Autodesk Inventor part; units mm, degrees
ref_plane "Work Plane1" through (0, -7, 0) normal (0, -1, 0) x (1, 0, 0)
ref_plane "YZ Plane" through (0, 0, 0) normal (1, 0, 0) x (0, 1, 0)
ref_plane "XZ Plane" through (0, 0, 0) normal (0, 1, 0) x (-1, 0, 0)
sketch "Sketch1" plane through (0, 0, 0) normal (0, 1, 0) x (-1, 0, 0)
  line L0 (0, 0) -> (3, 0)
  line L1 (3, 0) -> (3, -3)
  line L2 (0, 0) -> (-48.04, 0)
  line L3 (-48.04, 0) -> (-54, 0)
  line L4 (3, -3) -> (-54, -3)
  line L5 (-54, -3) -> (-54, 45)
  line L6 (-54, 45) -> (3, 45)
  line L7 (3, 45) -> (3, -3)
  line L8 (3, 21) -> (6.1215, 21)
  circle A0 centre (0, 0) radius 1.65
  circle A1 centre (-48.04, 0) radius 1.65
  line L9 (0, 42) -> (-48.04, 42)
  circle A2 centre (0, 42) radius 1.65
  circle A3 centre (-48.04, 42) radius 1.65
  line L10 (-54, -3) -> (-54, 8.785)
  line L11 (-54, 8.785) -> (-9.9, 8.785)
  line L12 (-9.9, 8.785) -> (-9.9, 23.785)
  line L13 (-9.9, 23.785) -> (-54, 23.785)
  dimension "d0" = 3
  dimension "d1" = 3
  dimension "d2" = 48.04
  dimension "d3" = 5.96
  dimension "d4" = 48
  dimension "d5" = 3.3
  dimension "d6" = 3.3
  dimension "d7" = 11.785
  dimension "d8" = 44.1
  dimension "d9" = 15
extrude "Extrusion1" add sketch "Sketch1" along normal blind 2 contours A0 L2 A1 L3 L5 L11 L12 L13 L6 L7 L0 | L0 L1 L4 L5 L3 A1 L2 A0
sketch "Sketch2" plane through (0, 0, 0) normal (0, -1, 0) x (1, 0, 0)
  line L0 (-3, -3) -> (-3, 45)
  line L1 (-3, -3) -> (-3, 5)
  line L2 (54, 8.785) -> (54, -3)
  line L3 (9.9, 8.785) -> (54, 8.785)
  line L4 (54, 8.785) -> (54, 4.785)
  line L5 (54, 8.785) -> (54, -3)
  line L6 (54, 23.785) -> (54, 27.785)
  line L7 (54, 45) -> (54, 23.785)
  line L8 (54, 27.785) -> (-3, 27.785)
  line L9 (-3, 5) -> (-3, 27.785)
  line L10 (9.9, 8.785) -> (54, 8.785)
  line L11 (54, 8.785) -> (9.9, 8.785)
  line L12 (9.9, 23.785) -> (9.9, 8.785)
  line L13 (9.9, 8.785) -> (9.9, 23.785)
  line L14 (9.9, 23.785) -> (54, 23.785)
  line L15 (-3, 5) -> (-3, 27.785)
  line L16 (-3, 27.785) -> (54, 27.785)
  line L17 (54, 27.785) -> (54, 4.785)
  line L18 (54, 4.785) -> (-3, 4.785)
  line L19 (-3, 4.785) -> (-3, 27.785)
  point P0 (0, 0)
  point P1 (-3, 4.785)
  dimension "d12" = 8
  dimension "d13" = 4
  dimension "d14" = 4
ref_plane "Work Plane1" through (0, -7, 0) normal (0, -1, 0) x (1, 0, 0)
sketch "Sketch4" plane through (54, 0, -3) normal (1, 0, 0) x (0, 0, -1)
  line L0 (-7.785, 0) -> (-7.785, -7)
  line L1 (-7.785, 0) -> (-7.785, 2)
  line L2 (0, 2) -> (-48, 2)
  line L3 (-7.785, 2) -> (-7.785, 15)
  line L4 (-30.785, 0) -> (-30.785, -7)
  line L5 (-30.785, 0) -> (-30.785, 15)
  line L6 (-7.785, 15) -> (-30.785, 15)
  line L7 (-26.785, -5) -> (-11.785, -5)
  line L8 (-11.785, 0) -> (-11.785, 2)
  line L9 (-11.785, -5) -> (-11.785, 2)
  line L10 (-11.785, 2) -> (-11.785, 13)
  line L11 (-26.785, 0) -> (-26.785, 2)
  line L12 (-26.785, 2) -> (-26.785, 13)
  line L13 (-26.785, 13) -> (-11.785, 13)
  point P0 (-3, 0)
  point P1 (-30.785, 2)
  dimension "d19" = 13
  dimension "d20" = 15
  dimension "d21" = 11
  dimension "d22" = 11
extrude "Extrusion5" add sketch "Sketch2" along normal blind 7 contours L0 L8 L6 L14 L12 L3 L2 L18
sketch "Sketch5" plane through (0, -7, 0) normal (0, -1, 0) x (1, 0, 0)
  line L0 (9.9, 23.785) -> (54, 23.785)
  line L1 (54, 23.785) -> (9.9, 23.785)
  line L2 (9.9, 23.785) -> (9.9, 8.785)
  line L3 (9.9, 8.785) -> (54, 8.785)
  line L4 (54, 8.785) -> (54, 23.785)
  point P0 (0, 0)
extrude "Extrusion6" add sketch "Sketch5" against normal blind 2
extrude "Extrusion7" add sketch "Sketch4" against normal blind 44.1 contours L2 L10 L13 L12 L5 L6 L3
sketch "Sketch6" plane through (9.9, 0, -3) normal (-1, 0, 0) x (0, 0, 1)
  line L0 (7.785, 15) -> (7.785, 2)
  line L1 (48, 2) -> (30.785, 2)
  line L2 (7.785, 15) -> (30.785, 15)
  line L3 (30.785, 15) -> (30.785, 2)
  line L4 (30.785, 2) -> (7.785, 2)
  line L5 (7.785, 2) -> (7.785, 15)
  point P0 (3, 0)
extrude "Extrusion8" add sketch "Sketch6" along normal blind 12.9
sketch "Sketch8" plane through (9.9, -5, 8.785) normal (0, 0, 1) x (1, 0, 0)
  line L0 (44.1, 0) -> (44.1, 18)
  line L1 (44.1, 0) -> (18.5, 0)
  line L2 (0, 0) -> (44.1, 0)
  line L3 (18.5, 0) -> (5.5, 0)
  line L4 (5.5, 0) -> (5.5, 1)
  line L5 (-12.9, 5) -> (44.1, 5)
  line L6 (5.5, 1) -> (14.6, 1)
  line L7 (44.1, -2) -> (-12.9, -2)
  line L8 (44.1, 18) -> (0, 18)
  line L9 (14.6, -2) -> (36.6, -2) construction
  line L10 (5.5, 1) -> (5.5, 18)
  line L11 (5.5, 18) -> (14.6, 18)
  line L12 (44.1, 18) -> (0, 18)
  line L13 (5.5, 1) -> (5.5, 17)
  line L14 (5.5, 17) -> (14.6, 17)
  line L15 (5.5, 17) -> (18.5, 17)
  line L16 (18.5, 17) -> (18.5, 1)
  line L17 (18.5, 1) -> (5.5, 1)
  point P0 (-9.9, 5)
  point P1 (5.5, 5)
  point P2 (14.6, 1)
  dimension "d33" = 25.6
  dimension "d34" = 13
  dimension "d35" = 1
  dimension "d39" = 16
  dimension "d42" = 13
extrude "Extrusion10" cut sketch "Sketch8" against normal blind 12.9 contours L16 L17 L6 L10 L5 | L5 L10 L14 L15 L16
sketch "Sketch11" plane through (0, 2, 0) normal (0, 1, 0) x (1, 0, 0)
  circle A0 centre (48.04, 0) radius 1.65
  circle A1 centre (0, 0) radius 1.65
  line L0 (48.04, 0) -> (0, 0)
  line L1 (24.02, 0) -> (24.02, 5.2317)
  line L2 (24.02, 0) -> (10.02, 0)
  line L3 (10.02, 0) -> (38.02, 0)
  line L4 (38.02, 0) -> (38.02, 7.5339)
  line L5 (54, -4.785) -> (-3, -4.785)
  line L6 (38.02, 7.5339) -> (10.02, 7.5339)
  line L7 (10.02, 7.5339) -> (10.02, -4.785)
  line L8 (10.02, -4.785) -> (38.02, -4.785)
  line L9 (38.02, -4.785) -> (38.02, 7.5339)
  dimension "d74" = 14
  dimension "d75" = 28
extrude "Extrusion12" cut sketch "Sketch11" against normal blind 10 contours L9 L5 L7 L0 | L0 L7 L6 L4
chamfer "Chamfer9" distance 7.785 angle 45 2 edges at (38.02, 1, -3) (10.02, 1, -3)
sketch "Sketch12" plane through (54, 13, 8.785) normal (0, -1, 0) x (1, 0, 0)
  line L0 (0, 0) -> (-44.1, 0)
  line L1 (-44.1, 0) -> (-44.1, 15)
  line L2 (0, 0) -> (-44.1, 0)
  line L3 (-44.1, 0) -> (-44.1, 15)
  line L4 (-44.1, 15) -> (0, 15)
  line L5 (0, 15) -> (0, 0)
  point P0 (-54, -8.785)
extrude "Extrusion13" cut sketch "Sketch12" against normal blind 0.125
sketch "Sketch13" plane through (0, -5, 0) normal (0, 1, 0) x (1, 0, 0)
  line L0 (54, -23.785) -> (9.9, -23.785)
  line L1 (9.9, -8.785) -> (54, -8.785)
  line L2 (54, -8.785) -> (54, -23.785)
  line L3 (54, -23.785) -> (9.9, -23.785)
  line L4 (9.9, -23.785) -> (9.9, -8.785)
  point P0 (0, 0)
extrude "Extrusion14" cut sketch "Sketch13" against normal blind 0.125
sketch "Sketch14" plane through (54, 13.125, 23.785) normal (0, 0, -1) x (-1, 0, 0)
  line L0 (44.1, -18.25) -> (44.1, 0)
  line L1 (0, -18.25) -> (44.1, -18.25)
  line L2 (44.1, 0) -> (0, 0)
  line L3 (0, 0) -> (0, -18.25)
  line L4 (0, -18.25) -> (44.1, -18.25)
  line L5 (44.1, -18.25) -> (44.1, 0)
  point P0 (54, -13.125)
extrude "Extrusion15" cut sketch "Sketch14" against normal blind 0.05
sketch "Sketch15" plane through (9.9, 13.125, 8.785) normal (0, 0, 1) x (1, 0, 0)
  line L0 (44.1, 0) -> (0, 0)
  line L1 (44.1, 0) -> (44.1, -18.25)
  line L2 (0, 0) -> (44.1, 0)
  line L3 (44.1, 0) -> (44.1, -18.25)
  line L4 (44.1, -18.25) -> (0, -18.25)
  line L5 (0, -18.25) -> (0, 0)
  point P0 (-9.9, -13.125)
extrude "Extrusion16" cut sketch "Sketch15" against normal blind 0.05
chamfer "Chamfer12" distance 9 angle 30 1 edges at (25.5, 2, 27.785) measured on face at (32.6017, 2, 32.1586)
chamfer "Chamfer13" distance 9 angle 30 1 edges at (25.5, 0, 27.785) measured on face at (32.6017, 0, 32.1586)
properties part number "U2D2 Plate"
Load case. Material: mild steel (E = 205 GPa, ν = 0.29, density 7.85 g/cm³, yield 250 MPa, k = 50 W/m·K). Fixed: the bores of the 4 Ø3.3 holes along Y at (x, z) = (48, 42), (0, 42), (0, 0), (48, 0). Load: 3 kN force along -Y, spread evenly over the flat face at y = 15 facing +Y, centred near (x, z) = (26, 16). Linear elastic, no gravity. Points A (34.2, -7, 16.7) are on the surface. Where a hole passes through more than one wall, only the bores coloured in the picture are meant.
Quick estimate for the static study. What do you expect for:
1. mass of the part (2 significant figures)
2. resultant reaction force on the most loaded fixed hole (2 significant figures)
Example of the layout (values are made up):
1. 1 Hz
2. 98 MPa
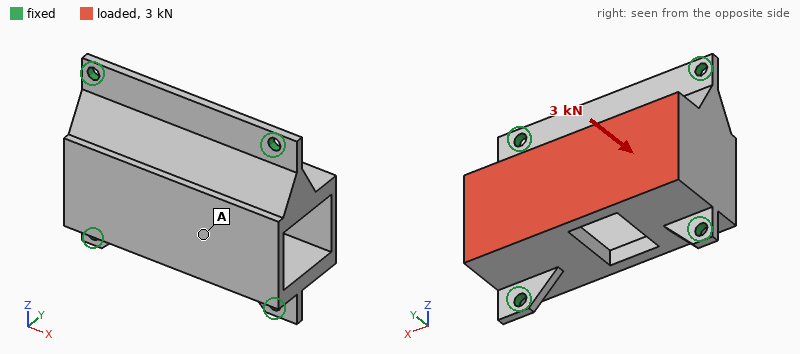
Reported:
1. 160 g
2. 970 N
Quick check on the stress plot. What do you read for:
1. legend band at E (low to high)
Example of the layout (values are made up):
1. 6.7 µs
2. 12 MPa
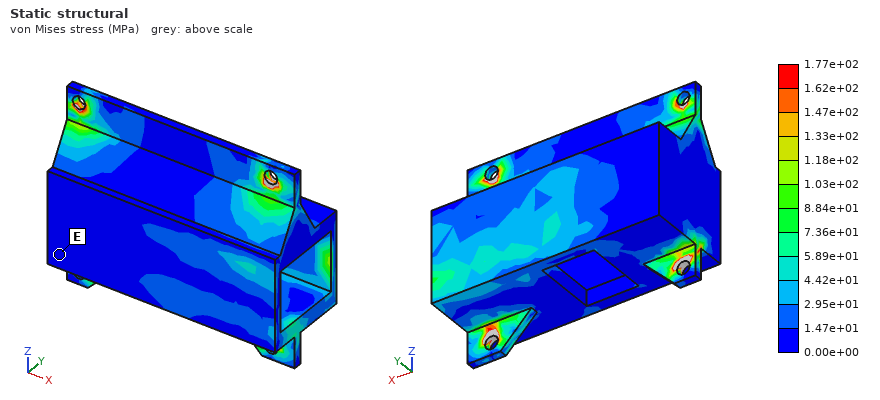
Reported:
1. 0.00e+00 to 1.47e+01 MPa
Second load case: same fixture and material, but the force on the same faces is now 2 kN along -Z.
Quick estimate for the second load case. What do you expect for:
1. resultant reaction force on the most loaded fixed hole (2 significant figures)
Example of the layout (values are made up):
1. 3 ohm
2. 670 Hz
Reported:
1. 730 N
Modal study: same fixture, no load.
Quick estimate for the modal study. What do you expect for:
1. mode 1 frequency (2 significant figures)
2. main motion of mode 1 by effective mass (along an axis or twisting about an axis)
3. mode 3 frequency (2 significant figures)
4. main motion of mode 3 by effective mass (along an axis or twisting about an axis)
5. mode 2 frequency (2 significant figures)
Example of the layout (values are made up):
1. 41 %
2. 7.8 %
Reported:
1. 6200 Hz
2. along Y
3. 10 kHz
4. along Z
5. 8000 Hz
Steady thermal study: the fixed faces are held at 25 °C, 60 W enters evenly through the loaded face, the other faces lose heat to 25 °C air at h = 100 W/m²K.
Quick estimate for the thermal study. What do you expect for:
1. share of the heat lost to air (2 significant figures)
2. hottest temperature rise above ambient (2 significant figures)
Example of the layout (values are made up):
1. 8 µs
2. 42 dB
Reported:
1. 60 %
2. 78 K
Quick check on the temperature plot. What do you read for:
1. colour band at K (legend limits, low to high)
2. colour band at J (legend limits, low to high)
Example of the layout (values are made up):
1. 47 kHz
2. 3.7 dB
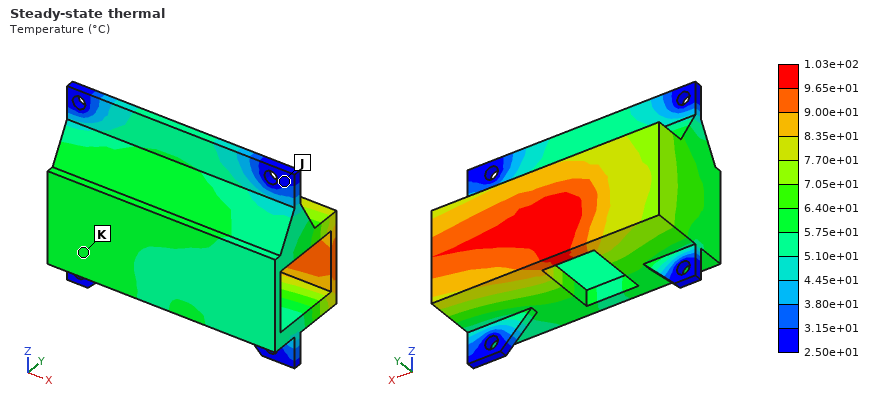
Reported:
1. 5.75e+01 to 6.40e+01 °C
2. 2.50e+01 to 3.15e+01 °C
